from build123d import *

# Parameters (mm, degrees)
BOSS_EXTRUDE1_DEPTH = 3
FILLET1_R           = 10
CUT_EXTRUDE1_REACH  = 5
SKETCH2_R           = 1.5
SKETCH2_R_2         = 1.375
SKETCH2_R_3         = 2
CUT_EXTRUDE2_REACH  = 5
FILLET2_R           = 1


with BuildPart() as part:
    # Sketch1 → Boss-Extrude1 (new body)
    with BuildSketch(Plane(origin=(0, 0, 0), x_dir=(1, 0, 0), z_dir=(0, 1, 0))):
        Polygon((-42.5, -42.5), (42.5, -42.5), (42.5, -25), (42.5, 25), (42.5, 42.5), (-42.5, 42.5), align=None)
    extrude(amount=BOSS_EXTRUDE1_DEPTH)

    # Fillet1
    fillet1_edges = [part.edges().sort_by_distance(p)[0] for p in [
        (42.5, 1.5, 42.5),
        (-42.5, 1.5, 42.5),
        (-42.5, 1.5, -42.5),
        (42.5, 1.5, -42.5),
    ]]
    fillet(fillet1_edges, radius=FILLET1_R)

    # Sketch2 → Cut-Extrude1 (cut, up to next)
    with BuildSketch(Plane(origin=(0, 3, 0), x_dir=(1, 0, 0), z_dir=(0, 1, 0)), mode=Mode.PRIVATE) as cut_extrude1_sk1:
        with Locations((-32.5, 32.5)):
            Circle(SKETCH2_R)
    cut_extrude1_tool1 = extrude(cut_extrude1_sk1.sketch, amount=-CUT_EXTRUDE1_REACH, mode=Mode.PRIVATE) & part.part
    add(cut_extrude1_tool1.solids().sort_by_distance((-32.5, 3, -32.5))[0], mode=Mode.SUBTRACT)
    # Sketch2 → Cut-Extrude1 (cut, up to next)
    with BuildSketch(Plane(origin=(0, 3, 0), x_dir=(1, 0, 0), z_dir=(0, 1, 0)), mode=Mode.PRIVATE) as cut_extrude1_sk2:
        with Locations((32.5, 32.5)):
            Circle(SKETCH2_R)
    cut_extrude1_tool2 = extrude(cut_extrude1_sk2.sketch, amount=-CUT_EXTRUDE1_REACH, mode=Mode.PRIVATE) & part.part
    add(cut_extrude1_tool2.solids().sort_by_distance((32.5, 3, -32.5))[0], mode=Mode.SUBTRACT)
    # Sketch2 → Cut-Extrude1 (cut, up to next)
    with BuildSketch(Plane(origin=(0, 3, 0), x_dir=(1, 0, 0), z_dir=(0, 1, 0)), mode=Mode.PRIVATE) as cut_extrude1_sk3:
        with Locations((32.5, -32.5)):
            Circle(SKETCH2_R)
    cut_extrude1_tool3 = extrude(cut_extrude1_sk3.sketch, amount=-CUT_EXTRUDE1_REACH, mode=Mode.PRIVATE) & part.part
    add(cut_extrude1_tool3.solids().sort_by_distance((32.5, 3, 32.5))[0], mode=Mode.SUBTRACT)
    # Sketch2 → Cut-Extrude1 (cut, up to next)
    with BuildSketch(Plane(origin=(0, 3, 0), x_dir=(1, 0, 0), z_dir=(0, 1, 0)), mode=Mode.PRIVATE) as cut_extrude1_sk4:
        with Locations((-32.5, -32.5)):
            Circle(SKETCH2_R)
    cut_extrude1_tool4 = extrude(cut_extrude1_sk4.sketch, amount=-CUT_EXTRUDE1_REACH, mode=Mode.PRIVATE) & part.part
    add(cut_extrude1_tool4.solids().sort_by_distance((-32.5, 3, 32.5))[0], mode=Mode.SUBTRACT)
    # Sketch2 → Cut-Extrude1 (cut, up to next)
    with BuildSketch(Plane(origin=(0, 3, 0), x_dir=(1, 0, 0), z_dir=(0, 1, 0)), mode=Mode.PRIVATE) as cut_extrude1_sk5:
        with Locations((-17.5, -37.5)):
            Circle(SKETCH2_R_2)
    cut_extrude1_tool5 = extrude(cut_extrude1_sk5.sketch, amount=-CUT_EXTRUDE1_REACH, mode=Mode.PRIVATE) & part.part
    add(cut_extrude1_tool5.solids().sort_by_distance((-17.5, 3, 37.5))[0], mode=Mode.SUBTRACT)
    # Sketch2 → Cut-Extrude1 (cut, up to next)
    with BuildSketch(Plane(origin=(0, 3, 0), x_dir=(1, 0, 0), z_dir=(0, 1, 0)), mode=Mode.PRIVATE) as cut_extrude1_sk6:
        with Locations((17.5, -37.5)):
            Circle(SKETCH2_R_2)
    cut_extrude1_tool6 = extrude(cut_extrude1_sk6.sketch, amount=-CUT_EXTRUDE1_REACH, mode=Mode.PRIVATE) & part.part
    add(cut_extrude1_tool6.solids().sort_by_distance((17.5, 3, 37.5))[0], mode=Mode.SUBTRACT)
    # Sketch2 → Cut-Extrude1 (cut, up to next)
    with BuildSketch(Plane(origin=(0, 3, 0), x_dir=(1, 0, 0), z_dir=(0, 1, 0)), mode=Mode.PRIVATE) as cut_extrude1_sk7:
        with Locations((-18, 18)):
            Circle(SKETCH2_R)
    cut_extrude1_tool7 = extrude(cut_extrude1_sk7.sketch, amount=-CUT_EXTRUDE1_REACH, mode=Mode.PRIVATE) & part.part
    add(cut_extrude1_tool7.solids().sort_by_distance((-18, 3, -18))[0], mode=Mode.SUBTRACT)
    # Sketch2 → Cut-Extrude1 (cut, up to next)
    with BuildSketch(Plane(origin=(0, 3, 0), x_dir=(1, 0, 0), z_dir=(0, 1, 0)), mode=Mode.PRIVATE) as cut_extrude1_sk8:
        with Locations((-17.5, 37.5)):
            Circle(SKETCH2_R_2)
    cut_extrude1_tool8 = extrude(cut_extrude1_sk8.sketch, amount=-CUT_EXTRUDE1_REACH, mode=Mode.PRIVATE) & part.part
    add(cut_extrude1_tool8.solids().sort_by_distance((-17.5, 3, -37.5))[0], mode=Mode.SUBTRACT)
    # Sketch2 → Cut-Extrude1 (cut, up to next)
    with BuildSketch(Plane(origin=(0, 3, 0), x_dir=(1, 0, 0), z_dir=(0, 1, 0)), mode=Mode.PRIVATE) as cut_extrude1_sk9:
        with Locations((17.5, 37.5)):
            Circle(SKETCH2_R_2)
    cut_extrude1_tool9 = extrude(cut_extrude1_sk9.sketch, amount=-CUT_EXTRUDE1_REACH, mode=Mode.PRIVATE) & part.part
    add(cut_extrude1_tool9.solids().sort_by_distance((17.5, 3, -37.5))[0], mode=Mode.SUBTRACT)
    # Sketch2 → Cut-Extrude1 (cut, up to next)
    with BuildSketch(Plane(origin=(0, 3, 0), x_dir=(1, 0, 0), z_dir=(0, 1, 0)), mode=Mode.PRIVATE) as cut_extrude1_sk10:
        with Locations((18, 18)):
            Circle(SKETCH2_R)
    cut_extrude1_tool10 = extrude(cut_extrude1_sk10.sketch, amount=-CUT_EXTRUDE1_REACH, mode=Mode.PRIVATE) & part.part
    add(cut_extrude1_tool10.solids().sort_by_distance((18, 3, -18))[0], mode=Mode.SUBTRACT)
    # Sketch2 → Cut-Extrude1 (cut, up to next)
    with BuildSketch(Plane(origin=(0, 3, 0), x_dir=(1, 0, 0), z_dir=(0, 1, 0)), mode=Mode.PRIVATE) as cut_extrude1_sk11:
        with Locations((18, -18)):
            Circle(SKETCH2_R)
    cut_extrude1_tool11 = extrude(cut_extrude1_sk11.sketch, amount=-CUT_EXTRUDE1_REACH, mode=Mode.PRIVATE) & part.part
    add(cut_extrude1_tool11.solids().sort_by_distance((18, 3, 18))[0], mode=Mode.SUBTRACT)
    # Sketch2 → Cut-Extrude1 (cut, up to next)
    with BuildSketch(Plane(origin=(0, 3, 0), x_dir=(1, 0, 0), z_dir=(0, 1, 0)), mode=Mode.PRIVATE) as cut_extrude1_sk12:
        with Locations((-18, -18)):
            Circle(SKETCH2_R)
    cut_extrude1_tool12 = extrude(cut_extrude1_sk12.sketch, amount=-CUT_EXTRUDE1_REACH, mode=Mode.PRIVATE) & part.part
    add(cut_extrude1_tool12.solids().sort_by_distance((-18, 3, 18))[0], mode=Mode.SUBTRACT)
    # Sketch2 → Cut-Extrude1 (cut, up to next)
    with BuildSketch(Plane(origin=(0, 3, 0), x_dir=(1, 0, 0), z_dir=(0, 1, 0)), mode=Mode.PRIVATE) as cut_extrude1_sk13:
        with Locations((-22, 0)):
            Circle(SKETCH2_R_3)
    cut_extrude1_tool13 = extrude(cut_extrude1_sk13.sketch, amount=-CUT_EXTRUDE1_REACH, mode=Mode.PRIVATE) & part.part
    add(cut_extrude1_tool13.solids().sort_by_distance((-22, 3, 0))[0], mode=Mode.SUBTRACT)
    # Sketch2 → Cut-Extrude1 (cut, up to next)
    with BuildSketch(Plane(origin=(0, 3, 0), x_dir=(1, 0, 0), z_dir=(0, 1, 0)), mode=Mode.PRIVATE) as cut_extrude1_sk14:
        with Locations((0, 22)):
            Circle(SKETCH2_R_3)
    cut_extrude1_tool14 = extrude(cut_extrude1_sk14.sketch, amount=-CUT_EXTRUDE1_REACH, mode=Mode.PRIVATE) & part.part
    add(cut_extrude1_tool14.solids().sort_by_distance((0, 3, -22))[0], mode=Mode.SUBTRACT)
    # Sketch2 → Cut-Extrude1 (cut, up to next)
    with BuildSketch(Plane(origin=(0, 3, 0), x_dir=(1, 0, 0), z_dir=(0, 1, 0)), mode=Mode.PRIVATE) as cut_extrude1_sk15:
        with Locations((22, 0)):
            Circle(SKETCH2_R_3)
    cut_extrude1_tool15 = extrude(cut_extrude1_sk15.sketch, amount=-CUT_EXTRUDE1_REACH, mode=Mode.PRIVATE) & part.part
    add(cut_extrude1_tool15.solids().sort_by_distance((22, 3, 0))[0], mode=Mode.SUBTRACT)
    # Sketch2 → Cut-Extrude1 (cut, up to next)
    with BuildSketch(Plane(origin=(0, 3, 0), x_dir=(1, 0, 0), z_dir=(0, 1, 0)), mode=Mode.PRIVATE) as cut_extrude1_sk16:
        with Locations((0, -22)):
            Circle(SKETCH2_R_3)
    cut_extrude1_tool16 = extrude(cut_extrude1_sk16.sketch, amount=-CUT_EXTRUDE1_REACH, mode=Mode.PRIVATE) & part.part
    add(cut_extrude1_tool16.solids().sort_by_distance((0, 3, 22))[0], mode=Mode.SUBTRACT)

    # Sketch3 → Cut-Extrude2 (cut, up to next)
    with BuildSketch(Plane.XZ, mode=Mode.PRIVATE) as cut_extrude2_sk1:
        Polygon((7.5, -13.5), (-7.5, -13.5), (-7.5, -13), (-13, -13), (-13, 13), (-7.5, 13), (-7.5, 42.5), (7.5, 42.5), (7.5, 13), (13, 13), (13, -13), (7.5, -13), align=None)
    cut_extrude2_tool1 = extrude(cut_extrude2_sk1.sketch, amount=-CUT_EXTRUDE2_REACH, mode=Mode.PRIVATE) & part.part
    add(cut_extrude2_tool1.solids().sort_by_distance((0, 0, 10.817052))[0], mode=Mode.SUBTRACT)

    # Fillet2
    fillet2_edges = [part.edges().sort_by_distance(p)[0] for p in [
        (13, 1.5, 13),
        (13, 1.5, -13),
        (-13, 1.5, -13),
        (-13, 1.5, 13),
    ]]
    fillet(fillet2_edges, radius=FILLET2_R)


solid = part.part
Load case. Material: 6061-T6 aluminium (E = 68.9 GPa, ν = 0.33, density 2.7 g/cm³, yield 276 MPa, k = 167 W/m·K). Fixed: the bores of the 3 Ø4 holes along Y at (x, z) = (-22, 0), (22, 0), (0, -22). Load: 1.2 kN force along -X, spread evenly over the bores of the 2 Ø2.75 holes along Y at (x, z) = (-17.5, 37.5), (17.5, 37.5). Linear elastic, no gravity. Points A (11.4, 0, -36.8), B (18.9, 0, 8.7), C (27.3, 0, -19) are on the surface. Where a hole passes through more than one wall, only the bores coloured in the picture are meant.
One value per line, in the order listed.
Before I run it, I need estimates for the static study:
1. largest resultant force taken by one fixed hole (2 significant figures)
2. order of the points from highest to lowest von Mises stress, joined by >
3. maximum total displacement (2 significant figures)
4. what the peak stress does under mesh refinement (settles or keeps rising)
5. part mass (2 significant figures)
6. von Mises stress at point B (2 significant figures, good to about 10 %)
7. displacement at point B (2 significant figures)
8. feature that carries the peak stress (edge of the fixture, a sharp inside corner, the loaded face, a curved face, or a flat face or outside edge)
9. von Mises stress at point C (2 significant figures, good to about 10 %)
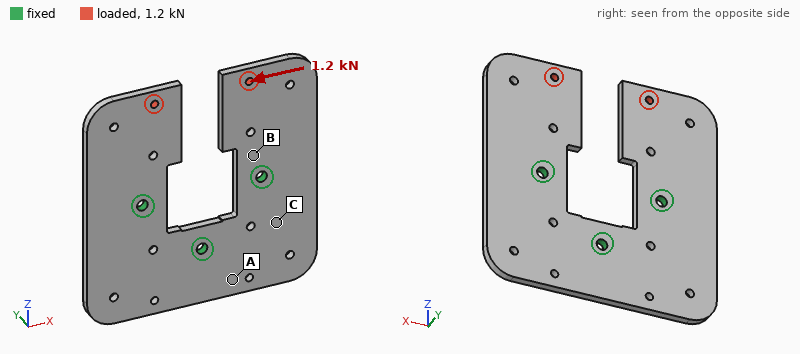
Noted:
1.3 kN
B > C > A
92 µm
keeps rising
48 g
25 MPa
15 µm
edge of the fixture
18 MPa
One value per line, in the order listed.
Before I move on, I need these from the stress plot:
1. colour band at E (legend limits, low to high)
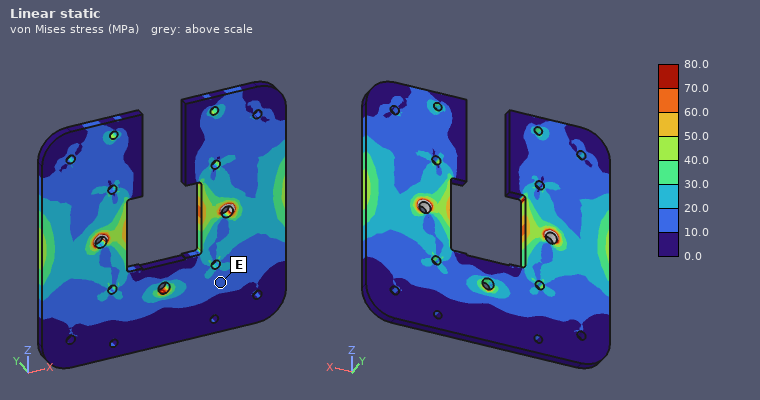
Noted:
10.0 to 20.0 MPa
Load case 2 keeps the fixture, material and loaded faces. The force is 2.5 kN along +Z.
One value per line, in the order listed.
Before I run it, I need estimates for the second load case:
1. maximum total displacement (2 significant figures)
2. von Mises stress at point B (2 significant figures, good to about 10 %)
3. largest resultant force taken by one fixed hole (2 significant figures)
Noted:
37 µm
31 MPa
1.2 kN
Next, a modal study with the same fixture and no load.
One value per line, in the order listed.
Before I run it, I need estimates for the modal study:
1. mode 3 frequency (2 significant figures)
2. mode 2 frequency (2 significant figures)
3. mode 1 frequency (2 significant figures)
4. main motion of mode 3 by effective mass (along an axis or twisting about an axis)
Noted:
2200 Hz
1200 Hz
1200 Hz
twisting about Z
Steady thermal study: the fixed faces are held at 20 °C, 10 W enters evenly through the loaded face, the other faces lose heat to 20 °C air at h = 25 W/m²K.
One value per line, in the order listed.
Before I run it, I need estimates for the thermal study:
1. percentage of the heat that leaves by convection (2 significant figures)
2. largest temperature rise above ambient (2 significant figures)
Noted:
14 %
16 K
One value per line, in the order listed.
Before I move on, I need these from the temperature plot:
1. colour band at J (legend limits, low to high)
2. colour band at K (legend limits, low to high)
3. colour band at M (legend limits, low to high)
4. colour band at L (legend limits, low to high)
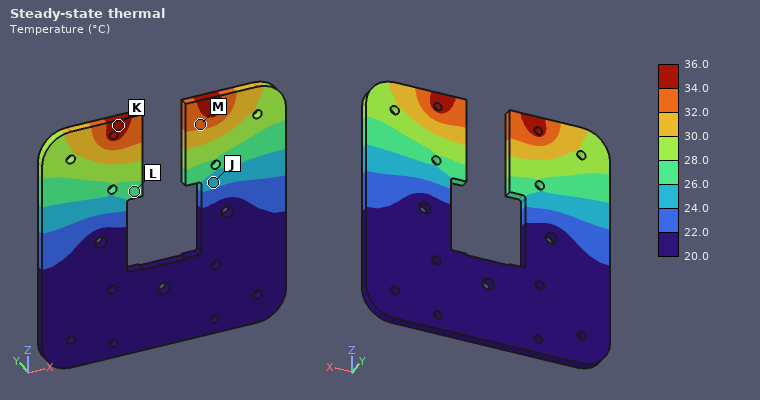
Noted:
24.0 to 26.0 °C
34.0 to 36.0 °C
32.0 to 34.0 °C
26.0 to 28.0 °C
